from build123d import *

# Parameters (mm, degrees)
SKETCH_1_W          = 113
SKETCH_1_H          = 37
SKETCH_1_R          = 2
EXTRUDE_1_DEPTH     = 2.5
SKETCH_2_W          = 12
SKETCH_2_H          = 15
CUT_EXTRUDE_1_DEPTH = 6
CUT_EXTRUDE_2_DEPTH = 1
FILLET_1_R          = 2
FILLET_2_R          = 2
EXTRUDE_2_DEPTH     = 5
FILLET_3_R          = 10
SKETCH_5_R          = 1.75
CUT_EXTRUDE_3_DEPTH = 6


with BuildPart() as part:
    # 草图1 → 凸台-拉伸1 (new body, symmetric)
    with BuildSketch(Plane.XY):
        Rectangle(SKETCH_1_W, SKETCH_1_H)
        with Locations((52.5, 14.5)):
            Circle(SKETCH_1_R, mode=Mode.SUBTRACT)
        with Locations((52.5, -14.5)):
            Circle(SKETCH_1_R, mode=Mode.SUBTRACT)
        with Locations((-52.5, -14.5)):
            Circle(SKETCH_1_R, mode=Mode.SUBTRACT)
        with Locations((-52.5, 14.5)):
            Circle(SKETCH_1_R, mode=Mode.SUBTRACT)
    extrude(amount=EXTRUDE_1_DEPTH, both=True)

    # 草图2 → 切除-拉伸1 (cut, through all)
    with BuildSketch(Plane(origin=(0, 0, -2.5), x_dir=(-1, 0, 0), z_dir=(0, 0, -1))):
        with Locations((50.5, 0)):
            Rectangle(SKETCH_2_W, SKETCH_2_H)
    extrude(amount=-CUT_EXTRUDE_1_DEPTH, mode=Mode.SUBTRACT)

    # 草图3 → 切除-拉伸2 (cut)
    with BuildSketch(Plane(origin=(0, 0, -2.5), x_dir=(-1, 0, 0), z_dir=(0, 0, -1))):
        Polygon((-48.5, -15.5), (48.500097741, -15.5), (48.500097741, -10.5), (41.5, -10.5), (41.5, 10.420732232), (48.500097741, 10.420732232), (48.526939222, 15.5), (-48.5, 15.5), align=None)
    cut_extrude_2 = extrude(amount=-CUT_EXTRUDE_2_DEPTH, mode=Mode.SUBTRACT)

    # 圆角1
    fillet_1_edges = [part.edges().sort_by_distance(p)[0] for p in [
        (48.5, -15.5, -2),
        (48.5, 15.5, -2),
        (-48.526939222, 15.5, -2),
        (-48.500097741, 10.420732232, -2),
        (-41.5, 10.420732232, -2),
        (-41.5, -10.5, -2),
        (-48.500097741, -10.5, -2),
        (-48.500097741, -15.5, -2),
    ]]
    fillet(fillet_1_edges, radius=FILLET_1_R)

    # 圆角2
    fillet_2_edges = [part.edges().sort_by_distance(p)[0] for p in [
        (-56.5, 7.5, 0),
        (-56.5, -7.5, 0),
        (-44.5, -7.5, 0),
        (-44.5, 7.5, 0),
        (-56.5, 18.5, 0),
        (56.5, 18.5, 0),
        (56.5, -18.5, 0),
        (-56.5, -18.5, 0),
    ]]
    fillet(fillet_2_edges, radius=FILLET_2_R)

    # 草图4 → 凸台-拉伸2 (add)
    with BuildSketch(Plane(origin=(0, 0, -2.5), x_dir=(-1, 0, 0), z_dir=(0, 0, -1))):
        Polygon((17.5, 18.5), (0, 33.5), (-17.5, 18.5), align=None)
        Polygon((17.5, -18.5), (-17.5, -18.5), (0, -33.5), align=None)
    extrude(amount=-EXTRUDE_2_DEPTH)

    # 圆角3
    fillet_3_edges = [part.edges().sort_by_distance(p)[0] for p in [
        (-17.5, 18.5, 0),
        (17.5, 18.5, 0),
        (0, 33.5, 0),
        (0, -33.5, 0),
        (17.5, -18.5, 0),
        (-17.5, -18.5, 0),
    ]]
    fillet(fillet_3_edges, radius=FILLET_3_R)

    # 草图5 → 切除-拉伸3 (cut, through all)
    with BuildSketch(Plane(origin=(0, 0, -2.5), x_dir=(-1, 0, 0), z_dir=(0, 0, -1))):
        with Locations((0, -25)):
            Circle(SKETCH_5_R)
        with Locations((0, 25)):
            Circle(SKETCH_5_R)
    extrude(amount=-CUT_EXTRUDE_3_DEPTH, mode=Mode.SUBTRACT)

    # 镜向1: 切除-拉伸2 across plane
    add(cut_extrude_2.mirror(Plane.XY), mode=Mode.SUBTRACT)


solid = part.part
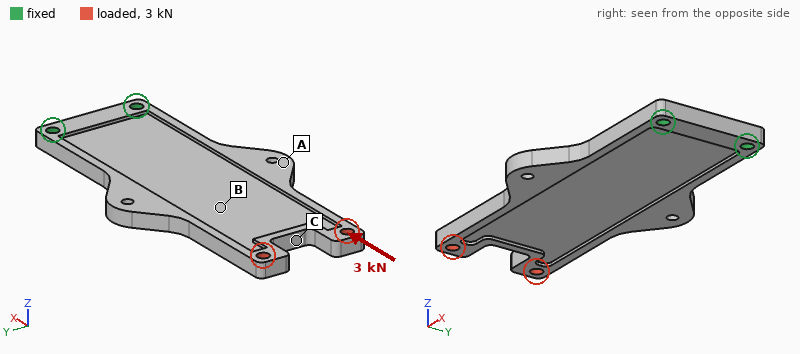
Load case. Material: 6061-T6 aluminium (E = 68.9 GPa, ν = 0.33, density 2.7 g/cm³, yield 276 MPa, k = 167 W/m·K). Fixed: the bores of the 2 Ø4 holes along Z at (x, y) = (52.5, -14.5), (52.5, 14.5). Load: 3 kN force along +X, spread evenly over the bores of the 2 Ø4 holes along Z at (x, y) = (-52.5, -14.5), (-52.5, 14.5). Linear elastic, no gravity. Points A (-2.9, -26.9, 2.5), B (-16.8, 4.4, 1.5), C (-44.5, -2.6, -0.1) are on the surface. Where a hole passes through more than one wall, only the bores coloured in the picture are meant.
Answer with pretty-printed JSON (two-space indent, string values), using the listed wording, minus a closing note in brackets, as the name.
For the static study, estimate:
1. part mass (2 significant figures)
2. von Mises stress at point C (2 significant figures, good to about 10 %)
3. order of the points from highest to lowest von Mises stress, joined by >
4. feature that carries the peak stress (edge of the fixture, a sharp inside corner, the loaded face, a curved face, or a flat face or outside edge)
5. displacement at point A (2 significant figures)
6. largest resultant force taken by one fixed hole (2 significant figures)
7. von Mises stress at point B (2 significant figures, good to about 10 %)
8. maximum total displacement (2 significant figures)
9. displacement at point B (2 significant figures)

{
  "part mass": "44 g",
  "von Mises stress at point C": "27 MPa",
  "order of the points from highest to lowest von Mises stress, joined by >": "C > B > A",
  "feature that carries the peak stress": "the loaded face",
  "displacement at point A": "19 µm",
  "largest resultant force taken by one fixed hole": "1.5 kN",
  "von Mises stress at point B": "18 MPa",
  "maximum total displacement": "49 µm",
  "displacement at point B": "24 µm"
}
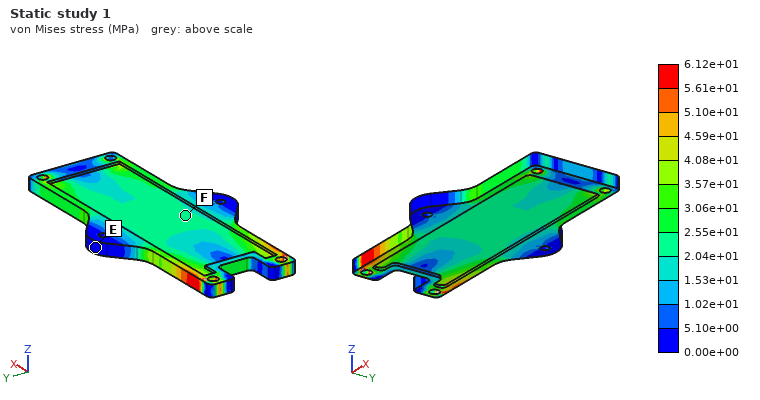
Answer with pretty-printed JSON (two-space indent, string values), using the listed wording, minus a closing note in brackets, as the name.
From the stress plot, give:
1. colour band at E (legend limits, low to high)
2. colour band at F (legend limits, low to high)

{
  "colour band at E": "0.00e+00 to 5.10e+00 MPa",
  "colour band at F": "2.04e+01 to 2.55e+01 MPa"
}
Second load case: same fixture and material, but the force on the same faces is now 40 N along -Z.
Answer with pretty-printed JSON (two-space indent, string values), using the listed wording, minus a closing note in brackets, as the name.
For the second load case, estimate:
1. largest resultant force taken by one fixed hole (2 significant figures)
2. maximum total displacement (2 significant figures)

{
  "largest resultant force taken by one fixed hole": "20 N",
  "maximum total displacement": "1.5 mm"
}
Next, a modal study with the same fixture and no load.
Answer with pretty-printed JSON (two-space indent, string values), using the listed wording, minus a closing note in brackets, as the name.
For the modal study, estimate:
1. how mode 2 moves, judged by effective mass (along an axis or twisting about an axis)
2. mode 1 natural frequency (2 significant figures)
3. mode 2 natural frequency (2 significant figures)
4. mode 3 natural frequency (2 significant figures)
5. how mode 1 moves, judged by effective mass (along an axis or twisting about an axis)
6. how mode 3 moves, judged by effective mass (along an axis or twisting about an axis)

{
  "how mode 2 moves, judged by effective mass": "twisting about X",
  "mode 1 natural frequency": "270 Hz",
  "mode 2 natural frequency": "1100 Hz",
  "mode 3 natural frequency": "1600 Hz",
  "how mode 1 moves, judged by effective mass": "along Z",
  "how mode 3 moves, judged by effective mass": "along Z"
}
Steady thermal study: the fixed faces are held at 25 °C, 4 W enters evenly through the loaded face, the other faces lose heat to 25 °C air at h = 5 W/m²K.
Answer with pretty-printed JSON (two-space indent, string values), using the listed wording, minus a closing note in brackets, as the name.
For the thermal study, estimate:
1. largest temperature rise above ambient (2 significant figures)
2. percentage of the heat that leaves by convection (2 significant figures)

{
  "largest temperature rise above ambient": "19 K",
  "percentage of the heat that leaves by convection": "12 %"
}
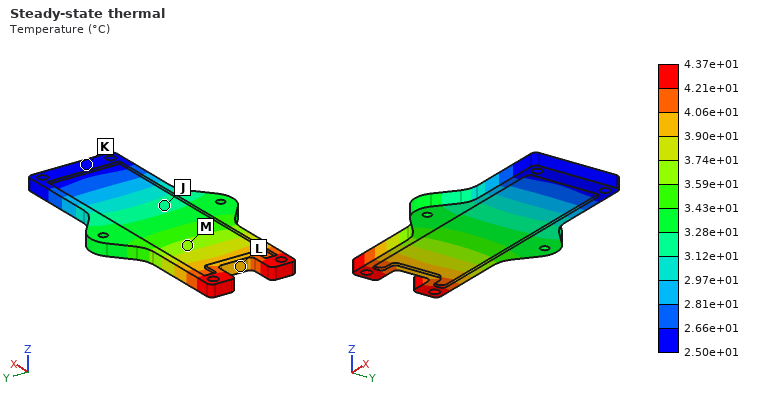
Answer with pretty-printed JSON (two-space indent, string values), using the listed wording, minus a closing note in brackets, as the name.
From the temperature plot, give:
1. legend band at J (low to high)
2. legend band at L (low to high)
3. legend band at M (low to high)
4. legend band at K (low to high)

{
  "legend band at J": "3.12e+01 to 3.28e+01 °C",
  "legend band at L": "3.90e+01 to 4.06e+01 °C",
  "legend band at M": "3.59e+01 to 3.74e+01 °C",
  "legend band at K": "2.50e+01 to 2.66e+01 °C"
}
